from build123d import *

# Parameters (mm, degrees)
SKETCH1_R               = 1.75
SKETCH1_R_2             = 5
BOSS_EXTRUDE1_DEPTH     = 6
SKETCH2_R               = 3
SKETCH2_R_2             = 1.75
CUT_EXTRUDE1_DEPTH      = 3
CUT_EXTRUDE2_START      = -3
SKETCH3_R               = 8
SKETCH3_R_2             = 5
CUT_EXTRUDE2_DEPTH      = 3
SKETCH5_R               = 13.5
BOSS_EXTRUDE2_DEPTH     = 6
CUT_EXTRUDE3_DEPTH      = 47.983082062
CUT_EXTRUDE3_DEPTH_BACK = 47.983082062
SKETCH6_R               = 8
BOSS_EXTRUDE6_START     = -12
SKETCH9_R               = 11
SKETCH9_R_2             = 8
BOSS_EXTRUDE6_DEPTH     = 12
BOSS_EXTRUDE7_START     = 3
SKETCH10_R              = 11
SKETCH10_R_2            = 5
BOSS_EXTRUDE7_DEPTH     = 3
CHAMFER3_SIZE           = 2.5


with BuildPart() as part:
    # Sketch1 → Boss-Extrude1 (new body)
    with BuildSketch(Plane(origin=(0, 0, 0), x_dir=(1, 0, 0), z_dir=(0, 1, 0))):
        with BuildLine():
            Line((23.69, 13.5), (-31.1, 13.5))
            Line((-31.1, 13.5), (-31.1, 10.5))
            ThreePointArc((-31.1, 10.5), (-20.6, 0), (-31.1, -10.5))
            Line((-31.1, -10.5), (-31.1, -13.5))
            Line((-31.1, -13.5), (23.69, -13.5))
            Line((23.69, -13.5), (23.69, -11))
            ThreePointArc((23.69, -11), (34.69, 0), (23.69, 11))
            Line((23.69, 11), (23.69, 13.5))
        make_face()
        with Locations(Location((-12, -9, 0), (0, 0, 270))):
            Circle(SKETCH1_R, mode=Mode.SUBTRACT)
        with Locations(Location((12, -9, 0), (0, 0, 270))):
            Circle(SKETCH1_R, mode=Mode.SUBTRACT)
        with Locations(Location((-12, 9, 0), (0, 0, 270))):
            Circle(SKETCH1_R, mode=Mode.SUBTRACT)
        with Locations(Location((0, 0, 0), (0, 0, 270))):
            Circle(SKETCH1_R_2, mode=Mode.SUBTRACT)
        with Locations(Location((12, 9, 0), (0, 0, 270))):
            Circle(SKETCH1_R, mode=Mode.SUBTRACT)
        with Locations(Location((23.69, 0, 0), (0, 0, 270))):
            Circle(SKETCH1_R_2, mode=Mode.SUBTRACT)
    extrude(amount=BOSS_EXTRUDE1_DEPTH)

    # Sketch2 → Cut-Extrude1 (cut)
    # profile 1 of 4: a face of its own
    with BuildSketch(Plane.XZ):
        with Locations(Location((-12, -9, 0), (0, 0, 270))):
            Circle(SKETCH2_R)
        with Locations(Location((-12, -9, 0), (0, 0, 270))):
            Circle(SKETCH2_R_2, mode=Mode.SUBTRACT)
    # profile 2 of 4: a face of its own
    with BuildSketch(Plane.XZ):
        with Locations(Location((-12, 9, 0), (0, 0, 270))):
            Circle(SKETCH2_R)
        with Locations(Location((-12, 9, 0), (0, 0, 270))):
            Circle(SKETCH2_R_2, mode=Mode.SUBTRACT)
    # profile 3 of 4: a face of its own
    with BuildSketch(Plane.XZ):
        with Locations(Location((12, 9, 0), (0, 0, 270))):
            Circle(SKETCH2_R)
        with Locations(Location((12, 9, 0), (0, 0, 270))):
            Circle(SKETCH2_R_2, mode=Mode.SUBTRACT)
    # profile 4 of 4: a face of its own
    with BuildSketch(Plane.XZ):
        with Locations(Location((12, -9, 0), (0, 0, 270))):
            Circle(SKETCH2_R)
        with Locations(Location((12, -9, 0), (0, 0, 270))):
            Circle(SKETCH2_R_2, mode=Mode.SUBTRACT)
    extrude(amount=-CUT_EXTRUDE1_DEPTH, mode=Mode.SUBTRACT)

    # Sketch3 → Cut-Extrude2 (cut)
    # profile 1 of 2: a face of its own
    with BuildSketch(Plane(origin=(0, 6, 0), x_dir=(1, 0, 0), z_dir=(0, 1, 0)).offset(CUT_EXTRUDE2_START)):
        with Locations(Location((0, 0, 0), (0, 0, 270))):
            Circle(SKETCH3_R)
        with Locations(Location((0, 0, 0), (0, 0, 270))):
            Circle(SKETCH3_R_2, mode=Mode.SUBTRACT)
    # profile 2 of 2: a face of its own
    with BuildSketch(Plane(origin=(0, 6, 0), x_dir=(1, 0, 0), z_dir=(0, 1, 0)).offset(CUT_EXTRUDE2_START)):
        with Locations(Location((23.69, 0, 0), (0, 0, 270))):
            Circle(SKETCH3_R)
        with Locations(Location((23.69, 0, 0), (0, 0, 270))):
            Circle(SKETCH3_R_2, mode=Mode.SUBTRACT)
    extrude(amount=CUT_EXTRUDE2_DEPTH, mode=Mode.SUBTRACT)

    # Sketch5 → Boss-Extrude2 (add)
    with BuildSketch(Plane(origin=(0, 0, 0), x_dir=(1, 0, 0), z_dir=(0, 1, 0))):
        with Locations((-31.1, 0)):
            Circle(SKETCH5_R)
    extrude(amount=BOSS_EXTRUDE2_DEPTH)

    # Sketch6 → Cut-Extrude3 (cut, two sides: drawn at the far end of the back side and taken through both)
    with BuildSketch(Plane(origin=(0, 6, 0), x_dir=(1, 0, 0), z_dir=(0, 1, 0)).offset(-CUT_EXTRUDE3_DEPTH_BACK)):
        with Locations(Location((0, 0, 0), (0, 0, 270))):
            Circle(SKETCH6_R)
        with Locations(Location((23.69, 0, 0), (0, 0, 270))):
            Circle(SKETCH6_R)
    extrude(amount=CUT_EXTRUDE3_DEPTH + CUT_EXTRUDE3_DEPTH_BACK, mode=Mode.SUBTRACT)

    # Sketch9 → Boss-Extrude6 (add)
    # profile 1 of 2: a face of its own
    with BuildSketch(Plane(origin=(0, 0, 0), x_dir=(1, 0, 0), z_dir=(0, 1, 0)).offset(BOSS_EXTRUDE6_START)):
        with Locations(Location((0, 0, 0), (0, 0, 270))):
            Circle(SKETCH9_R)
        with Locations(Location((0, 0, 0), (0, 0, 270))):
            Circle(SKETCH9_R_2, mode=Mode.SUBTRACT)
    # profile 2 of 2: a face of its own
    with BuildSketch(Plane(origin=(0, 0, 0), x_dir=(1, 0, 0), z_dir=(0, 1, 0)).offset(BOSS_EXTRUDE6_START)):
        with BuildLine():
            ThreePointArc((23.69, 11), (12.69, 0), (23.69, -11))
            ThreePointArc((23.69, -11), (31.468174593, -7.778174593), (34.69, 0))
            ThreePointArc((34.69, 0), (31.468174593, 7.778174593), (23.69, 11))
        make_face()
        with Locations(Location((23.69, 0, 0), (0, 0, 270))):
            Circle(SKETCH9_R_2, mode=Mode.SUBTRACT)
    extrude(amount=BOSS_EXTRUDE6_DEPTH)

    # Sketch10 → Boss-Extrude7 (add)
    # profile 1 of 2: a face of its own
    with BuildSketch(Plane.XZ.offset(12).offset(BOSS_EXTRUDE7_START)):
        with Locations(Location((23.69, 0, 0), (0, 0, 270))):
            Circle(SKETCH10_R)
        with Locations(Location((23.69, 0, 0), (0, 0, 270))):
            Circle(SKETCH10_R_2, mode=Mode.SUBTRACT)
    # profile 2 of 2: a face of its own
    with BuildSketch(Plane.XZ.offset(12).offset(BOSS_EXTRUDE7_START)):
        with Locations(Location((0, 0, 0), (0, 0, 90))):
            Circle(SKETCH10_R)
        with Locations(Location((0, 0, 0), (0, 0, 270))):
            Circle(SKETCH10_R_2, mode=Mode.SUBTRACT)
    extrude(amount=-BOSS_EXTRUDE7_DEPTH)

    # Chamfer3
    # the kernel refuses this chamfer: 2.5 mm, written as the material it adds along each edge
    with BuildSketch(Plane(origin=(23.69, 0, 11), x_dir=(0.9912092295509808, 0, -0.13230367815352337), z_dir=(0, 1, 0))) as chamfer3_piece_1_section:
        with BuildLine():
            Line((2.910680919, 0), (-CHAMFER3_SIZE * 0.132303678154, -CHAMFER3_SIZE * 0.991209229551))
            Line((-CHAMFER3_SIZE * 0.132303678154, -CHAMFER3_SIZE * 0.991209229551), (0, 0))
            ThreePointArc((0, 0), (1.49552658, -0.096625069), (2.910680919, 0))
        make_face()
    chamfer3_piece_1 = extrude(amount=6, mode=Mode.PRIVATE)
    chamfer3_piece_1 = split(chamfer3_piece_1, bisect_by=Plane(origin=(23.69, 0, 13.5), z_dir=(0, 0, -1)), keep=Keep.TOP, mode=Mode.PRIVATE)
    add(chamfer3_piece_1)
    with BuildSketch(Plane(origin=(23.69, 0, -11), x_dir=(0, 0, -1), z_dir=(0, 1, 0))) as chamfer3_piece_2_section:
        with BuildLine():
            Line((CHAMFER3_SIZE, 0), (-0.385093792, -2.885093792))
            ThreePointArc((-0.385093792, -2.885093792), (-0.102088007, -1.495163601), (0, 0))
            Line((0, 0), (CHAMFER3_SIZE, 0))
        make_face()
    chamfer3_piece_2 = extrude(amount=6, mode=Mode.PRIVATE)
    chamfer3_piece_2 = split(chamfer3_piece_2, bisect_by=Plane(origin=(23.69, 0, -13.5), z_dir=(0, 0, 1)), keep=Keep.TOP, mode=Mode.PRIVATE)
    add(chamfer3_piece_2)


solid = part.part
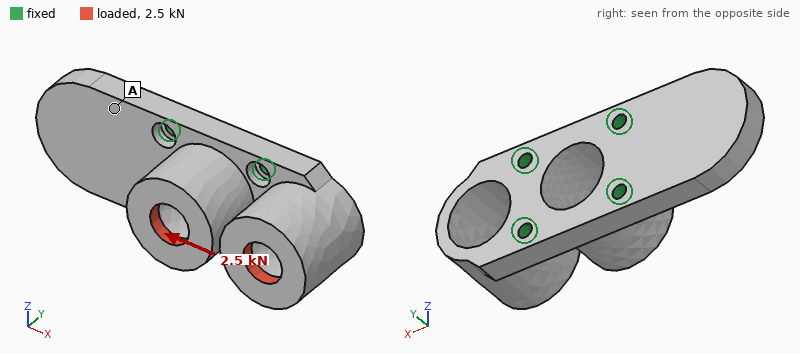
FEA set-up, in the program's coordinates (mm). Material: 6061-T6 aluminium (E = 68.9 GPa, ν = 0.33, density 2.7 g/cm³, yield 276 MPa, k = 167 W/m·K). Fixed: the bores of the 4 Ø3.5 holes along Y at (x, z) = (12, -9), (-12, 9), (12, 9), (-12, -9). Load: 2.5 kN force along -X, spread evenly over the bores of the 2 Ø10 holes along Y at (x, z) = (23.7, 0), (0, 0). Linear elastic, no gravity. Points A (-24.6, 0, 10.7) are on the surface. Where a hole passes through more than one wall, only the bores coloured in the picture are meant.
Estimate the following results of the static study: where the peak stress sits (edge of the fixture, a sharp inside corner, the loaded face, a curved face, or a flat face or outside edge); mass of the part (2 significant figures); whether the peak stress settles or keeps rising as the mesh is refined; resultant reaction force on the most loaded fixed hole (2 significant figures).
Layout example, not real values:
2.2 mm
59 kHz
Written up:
edge of the fixture
41 g
keeps rising
1.1 kN
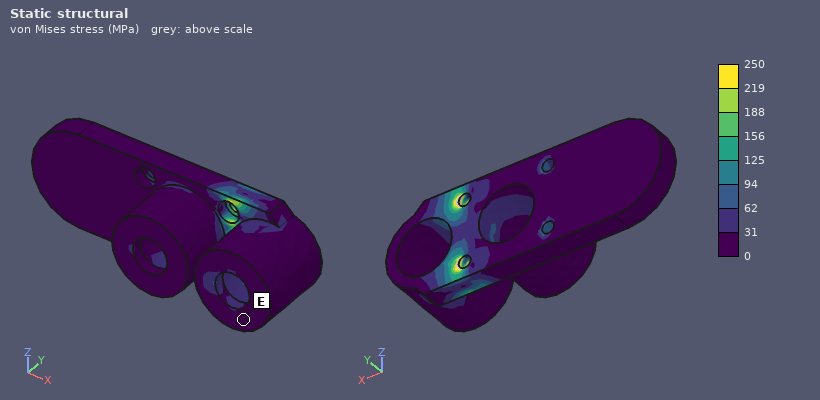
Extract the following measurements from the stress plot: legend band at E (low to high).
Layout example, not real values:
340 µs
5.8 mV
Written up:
0 to 31 MPa
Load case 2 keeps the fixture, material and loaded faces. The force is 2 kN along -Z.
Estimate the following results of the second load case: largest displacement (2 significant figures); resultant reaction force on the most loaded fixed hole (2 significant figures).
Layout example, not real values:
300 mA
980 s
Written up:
41 µm
1.7 kN
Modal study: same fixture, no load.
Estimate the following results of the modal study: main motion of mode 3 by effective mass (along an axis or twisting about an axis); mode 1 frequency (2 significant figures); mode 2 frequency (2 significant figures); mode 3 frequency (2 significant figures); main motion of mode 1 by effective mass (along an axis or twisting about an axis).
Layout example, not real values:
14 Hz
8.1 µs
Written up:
along Z
4200 Hz
4700 Hz
11 kHz
along Y
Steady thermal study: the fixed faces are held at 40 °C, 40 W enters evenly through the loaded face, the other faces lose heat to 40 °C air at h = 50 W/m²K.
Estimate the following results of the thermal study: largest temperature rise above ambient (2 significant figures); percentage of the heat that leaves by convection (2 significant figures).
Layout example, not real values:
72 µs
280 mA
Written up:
23 K
8.9 %
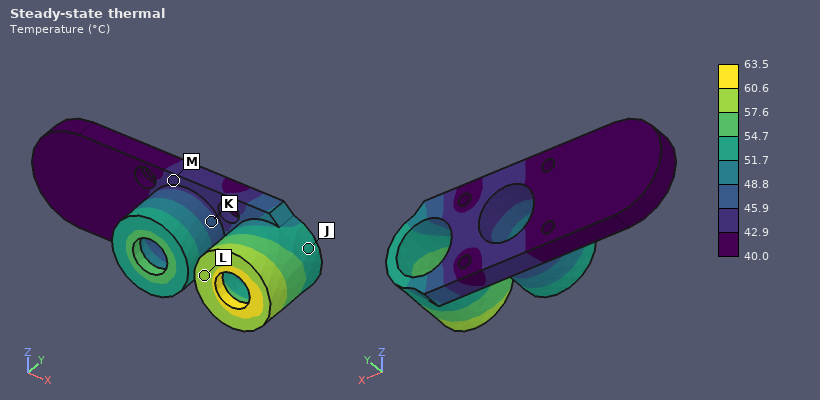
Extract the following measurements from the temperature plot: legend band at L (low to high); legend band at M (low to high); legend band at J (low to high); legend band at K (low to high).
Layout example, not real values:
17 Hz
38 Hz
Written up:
57.6 to 60.6 °C
42.9 to 45.9 °C
51.7 to 54.7 °C
45.9 to 48.8 °C
